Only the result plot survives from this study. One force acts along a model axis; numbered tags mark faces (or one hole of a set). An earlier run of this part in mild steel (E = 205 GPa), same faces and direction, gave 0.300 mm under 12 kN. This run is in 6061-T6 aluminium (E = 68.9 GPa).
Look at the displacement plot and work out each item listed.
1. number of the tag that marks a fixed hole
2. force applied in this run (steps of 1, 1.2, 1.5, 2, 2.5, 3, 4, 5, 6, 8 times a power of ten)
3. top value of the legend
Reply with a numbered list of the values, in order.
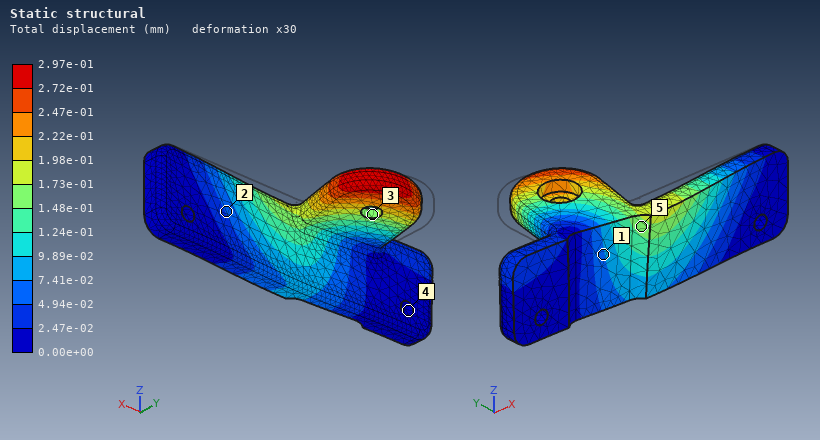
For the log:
1. 4
2. 4 kN
3. 2.97e-01 mm
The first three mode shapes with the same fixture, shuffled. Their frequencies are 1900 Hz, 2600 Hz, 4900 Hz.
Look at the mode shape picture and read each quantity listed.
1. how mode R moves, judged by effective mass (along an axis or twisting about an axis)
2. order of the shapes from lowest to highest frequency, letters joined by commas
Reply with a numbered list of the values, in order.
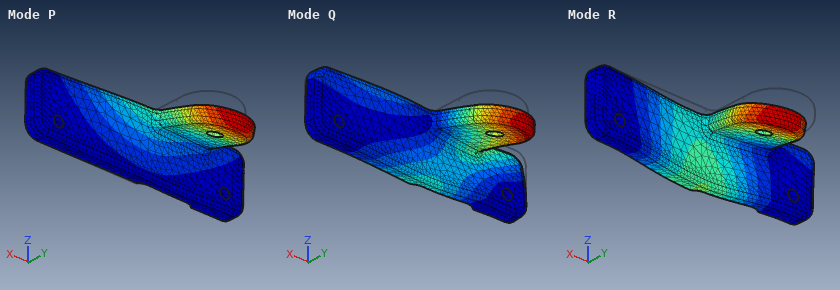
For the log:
1. along Y
2. P, R, Q
